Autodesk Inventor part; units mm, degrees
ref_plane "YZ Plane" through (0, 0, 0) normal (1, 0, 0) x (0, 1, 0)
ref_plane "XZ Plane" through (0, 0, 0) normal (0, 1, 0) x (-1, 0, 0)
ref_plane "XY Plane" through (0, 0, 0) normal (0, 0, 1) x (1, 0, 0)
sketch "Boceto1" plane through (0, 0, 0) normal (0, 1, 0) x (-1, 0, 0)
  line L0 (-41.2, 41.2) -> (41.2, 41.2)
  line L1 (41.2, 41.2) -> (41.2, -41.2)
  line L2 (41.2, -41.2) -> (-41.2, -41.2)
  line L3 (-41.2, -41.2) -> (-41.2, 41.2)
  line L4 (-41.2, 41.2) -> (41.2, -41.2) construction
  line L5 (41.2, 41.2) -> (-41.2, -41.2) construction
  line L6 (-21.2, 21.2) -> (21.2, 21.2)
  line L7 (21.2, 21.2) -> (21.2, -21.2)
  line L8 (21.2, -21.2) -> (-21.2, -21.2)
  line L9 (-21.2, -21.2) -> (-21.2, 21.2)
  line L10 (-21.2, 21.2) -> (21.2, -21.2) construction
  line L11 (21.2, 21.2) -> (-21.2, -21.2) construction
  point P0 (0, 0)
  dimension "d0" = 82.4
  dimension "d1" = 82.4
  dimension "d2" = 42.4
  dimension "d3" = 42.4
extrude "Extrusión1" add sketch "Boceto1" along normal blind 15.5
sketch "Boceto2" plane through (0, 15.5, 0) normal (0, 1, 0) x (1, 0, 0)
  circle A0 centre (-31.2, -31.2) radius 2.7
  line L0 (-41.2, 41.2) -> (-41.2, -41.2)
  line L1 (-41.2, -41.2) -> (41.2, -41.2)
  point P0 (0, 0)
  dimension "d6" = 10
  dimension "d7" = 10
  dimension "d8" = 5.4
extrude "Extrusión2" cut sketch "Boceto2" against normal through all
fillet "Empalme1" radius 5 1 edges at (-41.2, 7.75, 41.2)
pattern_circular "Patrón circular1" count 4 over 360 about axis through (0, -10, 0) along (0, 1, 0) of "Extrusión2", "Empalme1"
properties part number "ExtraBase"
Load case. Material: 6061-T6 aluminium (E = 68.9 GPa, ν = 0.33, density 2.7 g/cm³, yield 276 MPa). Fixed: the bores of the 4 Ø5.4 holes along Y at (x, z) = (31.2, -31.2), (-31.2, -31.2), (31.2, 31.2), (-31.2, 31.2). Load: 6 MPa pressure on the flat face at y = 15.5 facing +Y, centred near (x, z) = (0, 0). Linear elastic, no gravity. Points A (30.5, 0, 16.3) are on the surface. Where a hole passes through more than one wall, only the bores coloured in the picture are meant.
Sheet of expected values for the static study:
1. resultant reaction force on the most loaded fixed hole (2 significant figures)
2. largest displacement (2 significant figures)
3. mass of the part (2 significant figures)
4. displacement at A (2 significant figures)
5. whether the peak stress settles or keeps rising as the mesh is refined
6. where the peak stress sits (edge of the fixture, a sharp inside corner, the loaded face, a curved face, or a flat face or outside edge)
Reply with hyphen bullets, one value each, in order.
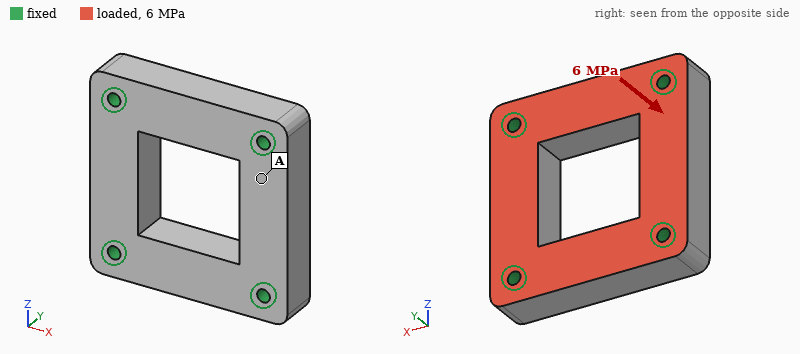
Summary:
- 7.3 kN
- 25 µm
- 200 g
- 14 µm
- keeps rising
- edge of the fixture
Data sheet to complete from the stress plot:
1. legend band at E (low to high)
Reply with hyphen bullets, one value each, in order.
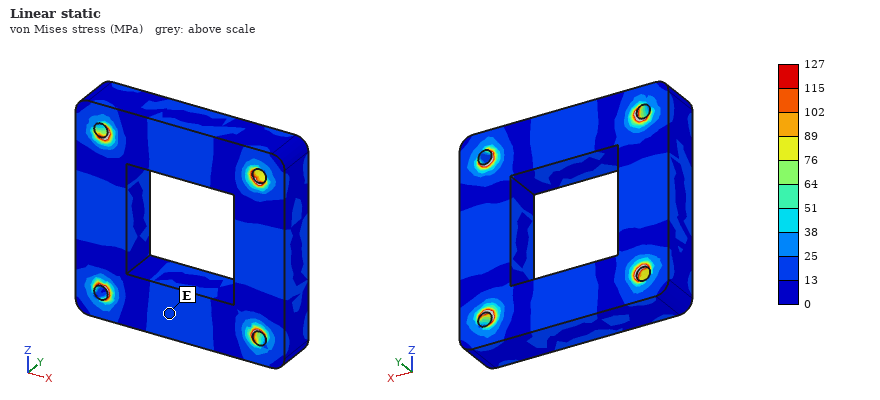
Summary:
- 13 to 25 MPa
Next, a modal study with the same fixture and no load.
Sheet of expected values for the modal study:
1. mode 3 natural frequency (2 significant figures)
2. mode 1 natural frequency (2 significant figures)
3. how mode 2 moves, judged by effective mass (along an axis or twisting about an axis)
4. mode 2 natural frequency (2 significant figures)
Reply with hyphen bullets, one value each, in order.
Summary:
- 15 kHz
- 13 kHz
- along Y
- 14 kHz
